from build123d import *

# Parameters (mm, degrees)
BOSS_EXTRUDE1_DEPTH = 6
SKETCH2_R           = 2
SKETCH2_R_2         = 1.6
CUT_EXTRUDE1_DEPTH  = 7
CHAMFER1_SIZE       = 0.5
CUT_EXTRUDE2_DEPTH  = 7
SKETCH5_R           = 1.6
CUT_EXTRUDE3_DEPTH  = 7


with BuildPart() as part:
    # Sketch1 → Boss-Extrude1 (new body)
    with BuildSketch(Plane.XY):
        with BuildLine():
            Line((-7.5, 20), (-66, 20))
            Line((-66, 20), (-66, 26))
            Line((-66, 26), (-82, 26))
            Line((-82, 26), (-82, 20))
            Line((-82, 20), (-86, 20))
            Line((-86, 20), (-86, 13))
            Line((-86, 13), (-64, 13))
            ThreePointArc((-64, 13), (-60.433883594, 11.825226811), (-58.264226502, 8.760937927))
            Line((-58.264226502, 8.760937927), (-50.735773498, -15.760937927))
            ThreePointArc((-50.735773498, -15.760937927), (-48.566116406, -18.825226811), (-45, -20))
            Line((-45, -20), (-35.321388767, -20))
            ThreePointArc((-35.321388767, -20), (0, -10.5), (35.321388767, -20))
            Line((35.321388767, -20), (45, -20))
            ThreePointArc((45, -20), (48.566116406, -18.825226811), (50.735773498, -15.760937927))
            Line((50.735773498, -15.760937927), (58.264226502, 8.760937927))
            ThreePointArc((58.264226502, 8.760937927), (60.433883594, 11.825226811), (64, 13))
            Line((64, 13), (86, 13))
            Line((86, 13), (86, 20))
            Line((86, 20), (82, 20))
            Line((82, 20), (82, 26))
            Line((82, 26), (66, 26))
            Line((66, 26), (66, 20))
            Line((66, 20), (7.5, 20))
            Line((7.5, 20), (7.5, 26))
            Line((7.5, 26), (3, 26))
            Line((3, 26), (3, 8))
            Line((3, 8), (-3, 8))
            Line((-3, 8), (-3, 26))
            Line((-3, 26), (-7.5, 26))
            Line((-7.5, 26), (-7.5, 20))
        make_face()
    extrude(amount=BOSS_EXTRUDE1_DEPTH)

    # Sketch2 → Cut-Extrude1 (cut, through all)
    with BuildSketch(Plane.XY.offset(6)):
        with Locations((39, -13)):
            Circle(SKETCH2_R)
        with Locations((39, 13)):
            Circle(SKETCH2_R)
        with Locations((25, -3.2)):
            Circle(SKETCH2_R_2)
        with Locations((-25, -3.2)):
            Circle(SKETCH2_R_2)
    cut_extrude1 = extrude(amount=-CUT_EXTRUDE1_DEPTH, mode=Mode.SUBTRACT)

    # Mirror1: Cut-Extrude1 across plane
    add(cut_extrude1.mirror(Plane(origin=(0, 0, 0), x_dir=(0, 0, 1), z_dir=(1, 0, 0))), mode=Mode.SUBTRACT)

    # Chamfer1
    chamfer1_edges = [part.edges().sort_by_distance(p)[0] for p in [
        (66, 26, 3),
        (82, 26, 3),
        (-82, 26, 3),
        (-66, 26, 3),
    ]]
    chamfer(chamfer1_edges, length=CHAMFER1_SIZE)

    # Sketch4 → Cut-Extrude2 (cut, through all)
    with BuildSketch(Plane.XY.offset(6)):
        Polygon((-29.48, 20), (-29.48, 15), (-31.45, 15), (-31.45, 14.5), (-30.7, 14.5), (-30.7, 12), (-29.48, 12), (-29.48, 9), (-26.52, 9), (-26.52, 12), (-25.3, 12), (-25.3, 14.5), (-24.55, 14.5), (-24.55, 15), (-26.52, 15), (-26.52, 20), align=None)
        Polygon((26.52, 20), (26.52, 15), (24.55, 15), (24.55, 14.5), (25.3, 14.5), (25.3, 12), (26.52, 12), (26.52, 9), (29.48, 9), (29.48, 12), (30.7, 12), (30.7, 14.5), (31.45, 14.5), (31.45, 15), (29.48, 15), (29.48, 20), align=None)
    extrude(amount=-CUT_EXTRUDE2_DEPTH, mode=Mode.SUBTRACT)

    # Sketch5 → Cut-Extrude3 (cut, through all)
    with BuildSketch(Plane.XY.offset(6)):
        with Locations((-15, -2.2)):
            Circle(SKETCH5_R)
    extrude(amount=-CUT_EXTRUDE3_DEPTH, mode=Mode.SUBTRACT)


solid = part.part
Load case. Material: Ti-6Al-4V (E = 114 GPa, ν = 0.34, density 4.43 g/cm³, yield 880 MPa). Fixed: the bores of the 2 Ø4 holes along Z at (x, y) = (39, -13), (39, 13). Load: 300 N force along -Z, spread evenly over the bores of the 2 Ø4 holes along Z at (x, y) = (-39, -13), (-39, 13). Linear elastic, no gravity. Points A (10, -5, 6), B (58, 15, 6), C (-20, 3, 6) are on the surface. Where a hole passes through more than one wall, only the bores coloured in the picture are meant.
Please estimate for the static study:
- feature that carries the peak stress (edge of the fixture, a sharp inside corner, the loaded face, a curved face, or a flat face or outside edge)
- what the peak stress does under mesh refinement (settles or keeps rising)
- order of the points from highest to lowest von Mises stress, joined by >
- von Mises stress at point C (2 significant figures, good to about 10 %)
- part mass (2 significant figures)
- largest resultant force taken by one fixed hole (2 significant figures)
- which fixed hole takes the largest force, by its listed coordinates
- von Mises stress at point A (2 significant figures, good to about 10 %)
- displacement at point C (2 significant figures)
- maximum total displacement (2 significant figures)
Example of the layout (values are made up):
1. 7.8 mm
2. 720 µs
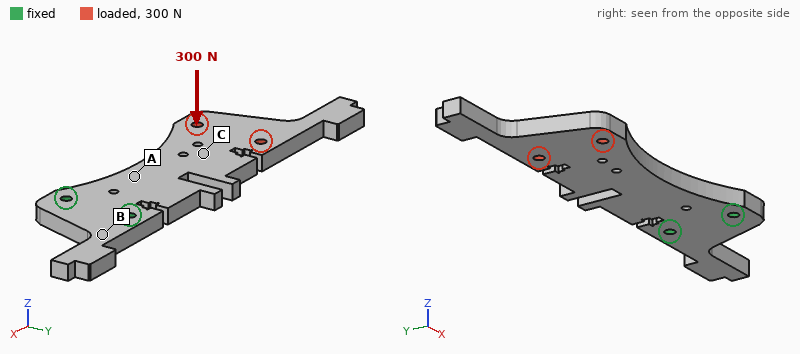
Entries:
1. edge of the fixture
2. keeps rising
3. A > C > B
4. 38 MPa
5. 120 g
6. 180 N
7. (39, -13)
8. 110 MPa
9. 0.61 mm
10. 1.8 mm
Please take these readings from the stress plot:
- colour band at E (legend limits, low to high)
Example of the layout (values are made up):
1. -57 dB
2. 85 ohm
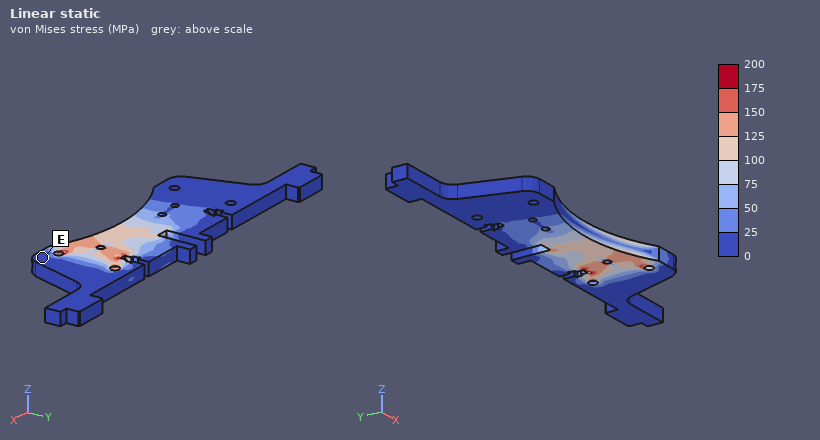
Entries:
1. 0 to 25 MPa
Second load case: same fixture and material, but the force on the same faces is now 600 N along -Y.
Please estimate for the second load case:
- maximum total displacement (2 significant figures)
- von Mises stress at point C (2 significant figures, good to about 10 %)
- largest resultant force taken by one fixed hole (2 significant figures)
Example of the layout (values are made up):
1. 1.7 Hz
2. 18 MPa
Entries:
1. 0.26 mm
2. 9.4 MPa
3. 1.8 kN
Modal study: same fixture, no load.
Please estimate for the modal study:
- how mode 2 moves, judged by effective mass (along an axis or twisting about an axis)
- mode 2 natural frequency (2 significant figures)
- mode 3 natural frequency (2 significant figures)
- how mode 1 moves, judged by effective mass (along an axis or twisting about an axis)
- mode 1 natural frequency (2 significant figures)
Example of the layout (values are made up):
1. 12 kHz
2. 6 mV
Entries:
1. along Y
2. 1300 Hz
3. 1700 Hz
4. along Z
5. 360 Hz
